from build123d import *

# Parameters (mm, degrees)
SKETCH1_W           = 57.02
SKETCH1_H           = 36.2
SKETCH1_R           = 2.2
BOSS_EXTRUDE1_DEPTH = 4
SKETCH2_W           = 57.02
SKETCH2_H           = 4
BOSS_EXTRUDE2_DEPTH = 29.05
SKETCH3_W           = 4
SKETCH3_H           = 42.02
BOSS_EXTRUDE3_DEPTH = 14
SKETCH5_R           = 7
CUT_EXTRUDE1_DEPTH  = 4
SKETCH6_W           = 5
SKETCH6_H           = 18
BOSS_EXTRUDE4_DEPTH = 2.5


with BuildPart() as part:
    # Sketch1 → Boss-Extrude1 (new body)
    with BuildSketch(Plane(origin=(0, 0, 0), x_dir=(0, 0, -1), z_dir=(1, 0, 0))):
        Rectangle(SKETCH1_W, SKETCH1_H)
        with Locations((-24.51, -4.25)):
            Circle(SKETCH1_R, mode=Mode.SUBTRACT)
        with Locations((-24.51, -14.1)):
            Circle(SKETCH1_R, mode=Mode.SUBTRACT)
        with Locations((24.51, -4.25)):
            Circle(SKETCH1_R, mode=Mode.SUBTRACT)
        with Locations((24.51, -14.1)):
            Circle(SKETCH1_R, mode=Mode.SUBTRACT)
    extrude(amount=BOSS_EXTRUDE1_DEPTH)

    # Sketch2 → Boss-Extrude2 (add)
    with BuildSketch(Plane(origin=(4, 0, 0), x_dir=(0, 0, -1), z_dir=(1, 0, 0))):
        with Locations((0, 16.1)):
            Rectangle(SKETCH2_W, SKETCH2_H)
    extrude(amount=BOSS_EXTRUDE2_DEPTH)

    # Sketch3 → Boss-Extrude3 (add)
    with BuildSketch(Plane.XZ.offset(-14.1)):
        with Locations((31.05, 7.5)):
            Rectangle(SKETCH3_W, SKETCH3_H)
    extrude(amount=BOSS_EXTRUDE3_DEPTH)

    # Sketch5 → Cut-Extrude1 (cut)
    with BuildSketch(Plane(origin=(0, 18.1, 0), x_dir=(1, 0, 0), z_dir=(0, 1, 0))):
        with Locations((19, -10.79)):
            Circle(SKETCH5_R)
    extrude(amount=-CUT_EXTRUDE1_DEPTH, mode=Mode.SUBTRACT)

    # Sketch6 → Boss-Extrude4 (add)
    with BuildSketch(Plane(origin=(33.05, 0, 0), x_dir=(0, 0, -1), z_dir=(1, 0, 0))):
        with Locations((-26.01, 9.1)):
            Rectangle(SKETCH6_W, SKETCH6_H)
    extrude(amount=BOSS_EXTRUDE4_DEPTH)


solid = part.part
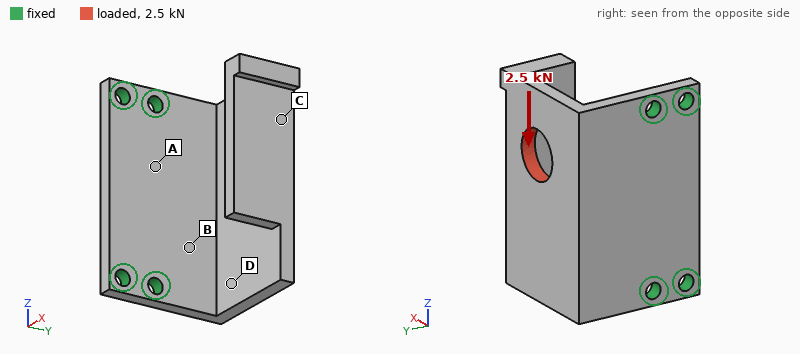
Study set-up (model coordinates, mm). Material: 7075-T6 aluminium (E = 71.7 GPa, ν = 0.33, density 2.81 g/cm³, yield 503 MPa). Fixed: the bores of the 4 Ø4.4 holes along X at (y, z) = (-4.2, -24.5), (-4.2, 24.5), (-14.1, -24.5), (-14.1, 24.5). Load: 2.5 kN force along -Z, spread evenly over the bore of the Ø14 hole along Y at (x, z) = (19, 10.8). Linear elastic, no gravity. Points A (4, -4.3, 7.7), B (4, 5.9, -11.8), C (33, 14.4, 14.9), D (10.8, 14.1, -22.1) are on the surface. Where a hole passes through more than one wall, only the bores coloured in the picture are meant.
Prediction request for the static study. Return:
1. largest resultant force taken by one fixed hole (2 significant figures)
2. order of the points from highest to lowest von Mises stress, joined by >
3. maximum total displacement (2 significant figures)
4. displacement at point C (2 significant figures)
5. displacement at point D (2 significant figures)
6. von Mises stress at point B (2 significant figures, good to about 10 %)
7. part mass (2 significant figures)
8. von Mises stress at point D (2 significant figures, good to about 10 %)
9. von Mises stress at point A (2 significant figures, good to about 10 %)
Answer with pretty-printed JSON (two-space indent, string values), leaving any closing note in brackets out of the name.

{
  "largest resultant force taken by one fixed hole": "1.7 kN",
  "order of the points from highest to lowest von Mises stress, joined by >": "B > D > A > C",
  "maximum total displacement": "0.41 mm",
  "displacement at point C": "0.28 mm",
  "displacement at point D": "0.18 mm",
  "von Mises stress at point B": "100 MPa",
  "part mass": "47 g",
  "von Mises stress at point D": "73 MPa",
  "von Mises stress at point A": "42 MPa"
}
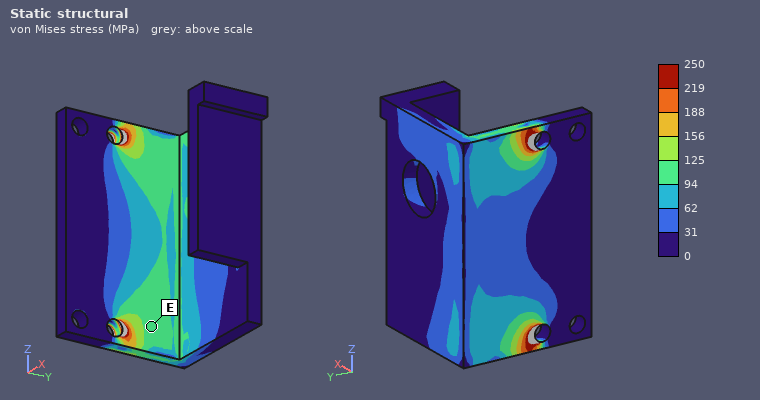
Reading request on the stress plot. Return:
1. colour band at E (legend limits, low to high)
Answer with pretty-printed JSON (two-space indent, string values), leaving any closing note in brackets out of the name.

{
  "colour band at E": "94 to 125 MPa"
}
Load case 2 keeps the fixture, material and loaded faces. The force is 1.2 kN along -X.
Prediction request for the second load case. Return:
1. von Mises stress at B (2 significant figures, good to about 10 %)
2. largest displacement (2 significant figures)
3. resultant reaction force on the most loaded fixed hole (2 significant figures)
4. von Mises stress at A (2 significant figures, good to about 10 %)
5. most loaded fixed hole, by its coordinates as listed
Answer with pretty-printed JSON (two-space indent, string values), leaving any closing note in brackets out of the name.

{
  "von Mises stress at B": "58 MPa",
  "largest displacement": "0.57 mm",
  "resultant reaction force on the most loaded fixed hole": "1.3 kN",
  "von Mises stress at A": "64 MPa",
  "most loaded fixed hole, by its coordinates as listed": "(-4.2, 24.5)"
}
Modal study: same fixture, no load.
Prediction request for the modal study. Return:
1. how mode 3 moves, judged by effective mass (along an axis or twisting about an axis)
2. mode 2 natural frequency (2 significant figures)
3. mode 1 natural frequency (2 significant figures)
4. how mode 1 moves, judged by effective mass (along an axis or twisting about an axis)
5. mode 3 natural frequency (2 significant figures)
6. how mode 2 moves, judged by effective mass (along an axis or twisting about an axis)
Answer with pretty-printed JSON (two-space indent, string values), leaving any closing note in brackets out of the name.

{
  "how mode 3 moves, judged by effective mass": "along X",
  "mode 2 natural frequency": "2200 Hz",
  "mode 1 natural frequency": "1200 Hz",
  "how mode 1 moves, judged by effective mass": "along Y",
  "mode 3 natural frequency": "2900 Hz",
  "how mode 2 moves, judged by effective mass": "along Z"
}
